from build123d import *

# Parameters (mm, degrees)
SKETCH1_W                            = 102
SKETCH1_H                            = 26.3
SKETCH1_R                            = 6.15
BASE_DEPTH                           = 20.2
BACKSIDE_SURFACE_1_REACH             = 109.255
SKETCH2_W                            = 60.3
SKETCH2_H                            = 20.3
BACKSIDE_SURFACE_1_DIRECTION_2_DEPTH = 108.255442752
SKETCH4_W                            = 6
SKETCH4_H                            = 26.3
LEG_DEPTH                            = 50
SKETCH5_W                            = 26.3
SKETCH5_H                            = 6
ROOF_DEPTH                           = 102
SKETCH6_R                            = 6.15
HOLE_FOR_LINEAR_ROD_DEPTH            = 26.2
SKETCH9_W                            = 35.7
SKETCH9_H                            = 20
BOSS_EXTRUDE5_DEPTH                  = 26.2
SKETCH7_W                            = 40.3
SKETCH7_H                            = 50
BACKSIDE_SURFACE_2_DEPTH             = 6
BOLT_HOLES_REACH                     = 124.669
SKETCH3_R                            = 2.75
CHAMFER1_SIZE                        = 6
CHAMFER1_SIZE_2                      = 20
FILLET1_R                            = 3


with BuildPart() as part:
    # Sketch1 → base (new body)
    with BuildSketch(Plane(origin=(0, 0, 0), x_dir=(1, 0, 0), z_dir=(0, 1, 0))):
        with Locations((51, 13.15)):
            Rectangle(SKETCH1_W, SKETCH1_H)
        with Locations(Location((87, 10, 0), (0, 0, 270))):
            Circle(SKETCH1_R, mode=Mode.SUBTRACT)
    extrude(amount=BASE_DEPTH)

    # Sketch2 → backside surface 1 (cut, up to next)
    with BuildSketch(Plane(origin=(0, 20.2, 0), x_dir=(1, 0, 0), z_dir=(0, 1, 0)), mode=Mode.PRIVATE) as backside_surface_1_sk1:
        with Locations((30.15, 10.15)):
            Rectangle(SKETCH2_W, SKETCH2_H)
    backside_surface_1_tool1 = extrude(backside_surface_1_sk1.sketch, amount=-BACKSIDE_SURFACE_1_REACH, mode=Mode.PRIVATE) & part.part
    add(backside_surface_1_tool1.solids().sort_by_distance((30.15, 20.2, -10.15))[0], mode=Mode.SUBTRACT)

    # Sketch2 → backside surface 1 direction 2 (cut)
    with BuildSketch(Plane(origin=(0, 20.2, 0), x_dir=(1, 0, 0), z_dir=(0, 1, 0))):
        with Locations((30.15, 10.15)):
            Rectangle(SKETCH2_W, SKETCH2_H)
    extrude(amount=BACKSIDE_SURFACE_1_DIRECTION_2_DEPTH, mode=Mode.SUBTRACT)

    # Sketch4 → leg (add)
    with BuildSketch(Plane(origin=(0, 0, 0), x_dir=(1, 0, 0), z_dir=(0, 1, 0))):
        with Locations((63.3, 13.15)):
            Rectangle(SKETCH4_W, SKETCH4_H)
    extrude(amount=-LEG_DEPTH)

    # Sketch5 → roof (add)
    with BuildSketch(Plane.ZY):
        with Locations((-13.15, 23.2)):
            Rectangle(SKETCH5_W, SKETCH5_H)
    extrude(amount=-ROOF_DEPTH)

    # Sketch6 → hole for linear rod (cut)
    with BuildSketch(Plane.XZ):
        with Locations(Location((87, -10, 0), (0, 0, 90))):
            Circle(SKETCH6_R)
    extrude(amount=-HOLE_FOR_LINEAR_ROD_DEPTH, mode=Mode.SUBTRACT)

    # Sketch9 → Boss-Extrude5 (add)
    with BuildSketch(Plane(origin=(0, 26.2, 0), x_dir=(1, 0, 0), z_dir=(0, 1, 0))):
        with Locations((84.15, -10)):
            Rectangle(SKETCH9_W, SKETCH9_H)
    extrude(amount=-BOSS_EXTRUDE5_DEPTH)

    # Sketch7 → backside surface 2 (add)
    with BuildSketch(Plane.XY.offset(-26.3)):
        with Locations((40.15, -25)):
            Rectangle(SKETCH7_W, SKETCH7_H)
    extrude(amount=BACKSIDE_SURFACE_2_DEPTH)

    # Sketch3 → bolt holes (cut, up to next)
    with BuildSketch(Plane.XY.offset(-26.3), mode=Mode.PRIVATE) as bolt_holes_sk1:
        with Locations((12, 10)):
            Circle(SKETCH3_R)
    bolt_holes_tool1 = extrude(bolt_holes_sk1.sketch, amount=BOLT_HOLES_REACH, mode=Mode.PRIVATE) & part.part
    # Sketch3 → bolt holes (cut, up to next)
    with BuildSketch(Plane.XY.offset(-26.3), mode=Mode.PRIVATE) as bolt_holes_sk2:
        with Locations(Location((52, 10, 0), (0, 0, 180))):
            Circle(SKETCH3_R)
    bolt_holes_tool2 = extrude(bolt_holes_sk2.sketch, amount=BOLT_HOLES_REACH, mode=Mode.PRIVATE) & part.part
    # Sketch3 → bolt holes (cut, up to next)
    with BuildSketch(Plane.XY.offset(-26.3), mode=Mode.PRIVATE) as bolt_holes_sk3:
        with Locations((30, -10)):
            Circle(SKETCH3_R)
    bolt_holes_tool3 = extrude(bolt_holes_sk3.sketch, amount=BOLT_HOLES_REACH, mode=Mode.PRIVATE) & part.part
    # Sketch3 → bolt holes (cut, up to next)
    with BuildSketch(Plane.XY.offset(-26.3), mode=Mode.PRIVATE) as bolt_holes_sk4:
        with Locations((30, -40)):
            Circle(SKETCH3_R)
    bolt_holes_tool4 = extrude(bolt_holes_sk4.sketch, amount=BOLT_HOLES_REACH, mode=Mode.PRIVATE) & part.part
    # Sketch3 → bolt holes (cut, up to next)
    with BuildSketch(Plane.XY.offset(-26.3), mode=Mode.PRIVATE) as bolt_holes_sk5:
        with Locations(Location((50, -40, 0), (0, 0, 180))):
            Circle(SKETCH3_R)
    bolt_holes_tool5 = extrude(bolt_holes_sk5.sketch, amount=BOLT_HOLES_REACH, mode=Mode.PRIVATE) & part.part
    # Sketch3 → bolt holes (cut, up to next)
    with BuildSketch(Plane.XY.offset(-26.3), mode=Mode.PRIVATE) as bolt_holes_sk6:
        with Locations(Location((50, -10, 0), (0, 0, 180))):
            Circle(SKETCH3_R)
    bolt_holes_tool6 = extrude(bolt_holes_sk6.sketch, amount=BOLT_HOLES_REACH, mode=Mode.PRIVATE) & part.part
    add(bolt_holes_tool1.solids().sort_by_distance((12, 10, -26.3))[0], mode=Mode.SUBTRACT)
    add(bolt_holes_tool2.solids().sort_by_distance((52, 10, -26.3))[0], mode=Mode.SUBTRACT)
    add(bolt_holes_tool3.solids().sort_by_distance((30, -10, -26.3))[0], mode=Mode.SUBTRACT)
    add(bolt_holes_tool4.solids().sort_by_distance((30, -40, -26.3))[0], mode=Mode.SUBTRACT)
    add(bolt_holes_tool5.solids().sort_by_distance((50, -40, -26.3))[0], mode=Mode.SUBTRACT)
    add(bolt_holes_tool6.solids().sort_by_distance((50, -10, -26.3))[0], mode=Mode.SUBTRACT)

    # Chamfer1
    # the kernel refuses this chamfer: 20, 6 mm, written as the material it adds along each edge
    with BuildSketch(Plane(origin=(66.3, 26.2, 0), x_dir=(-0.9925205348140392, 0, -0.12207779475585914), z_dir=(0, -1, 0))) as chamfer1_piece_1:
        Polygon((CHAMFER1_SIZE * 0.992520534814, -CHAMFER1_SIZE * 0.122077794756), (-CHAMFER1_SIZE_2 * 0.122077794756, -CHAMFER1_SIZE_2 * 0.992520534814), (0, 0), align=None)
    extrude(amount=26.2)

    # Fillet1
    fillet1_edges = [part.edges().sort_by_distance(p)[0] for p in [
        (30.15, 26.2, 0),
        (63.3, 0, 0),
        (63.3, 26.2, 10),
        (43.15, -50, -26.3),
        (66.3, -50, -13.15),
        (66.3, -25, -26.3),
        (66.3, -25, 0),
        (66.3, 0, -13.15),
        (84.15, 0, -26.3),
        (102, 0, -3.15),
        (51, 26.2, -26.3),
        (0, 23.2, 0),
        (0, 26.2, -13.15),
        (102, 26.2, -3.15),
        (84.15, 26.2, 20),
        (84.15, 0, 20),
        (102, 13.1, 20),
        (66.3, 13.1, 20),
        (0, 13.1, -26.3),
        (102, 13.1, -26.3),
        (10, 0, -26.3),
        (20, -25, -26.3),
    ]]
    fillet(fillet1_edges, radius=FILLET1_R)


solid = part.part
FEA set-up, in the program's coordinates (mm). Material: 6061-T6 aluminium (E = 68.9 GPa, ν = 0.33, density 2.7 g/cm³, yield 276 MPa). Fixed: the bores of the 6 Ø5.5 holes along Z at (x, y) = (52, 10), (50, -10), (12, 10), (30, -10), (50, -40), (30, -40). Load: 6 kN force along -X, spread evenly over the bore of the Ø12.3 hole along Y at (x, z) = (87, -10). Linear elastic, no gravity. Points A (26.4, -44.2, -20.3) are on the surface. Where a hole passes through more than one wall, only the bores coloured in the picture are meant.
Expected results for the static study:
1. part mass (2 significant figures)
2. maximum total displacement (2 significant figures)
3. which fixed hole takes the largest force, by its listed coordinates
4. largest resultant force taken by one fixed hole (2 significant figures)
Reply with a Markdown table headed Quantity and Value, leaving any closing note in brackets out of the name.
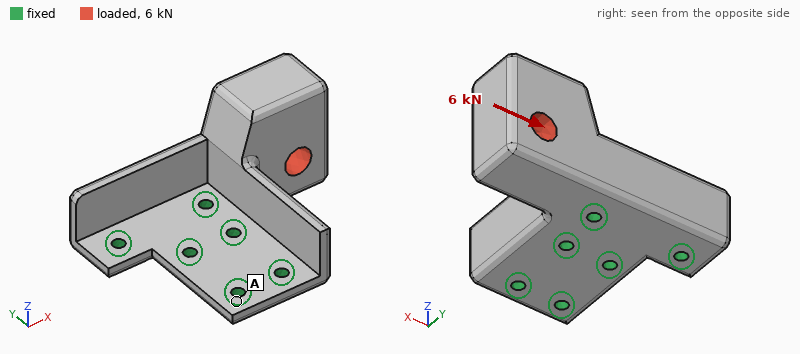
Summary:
| Quantity | Value |
|---|---|
| part mass | 220 g |
| maximum total displacement | 0.18 mm |
| which fixed hole takes the largest force, by its listed coordinates | (52, 10) |
| largest resultant force taken by one fixed hole | 3.6 kN |
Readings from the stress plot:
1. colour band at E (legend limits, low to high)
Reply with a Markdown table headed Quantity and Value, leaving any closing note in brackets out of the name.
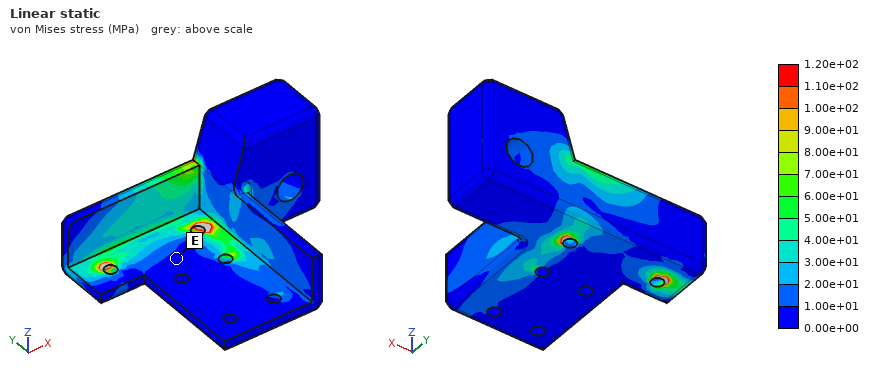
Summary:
| Quantity | Value |
|---|---|
| colour band at E | 0.00e+00 to 1.00e+01 MPa |
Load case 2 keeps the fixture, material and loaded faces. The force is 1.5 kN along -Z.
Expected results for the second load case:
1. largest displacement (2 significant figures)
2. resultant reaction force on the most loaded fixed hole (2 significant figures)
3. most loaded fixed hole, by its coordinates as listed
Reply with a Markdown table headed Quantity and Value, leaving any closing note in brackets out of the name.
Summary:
| Quantity | Value |
|---|---|
| largest displacement | 0.14 mm |
| resultant reaction force on the most loaded fixed hole | 2.6 kN |
| most loaded fixed hole, by its coordinates as listed | (52, 10) |
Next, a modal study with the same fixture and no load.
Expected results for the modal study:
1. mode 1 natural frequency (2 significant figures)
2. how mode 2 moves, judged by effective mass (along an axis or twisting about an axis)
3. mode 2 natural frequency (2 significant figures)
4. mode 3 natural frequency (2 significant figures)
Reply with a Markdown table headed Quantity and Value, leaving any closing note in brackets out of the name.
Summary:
| Quantity | Value |
|---|---|
| mode 1 natural frequency | 1800 Hz |
| how mode 2 moves, judged by effective mass | along Y |
| mode 2 natural frequency | 3700 Hz |
| mode 3 natural frequency | 5300 Hz |
